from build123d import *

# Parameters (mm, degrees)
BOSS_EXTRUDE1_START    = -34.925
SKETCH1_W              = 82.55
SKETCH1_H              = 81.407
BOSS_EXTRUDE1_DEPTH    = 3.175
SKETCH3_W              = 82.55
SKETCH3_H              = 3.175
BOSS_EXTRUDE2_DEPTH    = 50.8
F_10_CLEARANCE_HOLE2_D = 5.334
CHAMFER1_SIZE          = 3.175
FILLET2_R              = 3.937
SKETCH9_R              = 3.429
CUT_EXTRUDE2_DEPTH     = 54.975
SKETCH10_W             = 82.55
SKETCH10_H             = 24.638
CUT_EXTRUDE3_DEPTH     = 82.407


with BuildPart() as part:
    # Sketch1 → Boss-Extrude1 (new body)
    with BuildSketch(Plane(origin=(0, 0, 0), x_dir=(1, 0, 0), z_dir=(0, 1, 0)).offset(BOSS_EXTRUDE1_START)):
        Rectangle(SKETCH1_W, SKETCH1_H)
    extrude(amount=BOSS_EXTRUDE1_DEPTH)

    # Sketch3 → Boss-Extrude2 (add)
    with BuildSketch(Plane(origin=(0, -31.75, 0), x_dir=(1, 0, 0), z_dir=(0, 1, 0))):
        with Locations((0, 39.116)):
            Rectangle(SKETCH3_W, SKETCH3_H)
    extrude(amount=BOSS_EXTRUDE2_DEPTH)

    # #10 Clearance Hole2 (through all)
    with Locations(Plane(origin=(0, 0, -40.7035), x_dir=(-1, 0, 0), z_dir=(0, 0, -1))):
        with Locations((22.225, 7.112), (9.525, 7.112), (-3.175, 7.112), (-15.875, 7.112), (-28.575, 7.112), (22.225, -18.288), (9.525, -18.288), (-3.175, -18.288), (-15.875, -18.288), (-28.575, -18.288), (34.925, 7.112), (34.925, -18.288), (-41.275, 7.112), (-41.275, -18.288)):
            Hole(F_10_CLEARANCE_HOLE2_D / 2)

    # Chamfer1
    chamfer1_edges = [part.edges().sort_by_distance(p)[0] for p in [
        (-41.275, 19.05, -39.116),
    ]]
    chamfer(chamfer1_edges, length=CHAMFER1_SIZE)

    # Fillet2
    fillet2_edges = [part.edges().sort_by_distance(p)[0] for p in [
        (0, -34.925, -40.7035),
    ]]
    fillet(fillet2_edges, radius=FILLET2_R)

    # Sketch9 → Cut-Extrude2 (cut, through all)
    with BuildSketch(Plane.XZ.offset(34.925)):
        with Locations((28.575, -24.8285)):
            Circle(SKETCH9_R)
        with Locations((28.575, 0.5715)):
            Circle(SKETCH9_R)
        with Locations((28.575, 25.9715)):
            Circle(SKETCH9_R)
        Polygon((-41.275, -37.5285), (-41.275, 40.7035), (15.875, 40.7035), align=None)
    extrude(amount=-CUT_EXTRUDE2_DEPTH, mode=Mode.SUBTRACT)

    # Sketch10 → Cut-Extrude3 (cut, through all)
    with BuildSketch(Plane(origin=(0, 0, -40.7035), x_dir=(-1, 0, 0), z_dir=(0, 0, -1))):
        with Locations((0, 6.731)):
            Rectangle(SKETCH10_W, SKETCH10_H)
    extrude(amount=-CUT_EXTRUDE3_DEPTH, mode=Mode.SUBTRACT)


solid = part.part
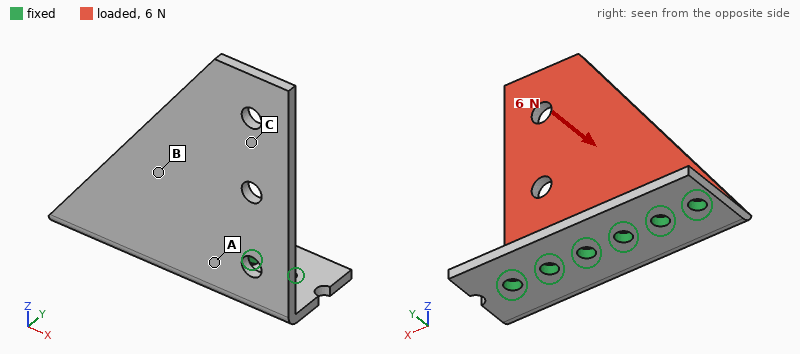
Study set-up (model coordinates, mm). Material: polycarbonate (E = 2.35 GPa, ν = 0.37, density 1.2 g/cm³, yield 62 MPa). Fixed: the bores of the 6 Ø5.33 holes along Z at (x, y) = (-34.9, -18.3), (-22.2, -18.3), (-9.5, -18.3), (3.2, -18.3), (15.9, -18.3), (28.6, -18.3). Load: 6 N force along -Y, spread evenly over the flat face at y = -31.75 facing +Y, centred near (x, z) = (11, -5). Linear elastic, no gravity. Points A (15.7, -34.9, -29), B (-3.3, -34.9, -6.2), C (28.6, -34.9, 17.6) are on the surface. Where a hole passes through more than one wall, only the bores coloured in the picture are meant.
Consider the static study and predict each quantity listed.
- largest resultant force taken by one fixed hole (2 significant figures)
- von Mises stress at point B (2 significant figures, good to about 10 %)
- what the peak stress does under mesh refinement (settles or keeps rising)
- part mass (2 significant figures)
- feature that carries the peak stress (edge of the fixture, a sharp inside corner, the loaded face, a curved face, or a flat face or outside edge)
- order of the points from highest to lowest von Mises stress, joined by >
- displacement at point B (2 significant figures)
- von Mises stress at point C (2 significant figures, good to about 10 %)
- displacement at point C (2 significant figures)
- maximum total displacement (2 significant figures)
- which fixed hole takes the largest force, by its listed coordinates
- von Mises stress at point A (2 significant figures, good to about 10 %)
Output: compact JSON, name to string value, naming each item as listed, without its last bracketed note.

{"largest resultant force taken by one fixed hole": "1.8 N", "von Mises stress at point B": "0.73 MPa", "what the peak stress does under mesh refinement": "keeps rising", "part mass": "24 g", "feature that carries the peak stress": "edge of the fixture", "order of the points from highest to lowest von Mises stress, joined by >": "A > B > C", "displacement at point B": "0.31 mm", "von Mises stress at point C": "0.24 MPa", "displacement at point C": "0.76 mm", "maximum total displacement": "1.2 mm", "which fixed hole takes the largest force, by its listed coordinates": "(28.6, -18.3)", "von Mises stress at point A": "1.2 MPa"}
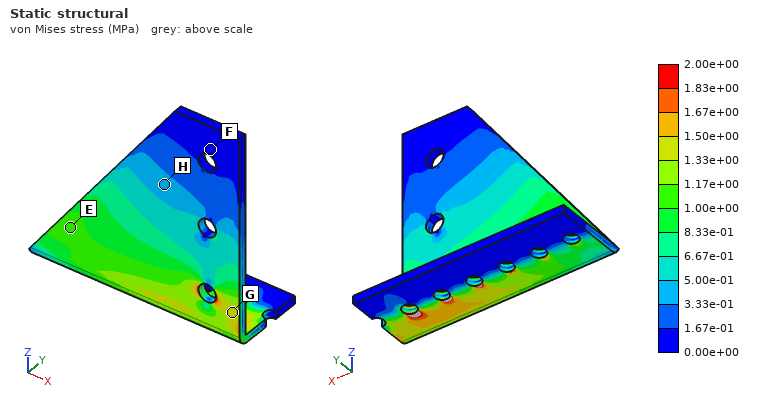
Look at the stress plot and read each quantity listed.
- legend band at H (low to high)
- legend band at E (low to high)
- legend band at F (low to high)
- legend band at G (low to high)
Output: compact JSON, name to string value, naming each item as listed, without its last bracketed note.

{"legend band at H": "3.33e-01 to 5.00e-01 MPa", "legend band at E": "1.00e+00 to 1.17e+00 MPa", "legend band at F": "0.00e+00 to 1.67e-01 MPa", "legend band at G": "1.33e+00 to 1.50e+00 MPa"}
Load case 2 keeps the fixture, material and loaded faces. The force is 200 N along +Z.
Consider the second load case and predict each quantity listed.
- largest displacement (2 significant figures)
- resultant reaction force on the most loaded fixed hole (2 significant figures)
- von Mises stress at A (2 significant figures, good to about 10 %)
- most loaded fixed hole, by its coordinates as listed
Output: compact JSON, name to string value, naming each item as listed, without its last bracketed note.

{"largest displacement": "1.2 mm", "resultant reaction force on the most loaded fixed hole": "70 N", "von Mises stress at A": "2.4 MPa", "most loaded fixed hole, by its coordinates as listed": "(28.6, -18.3)"}
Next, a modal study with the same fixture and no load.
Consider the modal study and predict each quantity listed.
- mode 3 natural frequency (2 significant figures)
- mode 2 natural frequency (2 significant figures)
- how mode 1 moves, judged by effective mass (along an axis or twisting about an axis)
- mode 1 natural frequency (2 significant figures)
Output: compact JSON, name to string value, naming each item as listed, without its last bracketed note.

{"mode 3 natural frequency": "570 Hz", "mode 2 natural frequency": "470 Hz", "how mode 1 moves, judged by effective mass": "along Y", "mode 1 natural frequency": "120 Hz"}
